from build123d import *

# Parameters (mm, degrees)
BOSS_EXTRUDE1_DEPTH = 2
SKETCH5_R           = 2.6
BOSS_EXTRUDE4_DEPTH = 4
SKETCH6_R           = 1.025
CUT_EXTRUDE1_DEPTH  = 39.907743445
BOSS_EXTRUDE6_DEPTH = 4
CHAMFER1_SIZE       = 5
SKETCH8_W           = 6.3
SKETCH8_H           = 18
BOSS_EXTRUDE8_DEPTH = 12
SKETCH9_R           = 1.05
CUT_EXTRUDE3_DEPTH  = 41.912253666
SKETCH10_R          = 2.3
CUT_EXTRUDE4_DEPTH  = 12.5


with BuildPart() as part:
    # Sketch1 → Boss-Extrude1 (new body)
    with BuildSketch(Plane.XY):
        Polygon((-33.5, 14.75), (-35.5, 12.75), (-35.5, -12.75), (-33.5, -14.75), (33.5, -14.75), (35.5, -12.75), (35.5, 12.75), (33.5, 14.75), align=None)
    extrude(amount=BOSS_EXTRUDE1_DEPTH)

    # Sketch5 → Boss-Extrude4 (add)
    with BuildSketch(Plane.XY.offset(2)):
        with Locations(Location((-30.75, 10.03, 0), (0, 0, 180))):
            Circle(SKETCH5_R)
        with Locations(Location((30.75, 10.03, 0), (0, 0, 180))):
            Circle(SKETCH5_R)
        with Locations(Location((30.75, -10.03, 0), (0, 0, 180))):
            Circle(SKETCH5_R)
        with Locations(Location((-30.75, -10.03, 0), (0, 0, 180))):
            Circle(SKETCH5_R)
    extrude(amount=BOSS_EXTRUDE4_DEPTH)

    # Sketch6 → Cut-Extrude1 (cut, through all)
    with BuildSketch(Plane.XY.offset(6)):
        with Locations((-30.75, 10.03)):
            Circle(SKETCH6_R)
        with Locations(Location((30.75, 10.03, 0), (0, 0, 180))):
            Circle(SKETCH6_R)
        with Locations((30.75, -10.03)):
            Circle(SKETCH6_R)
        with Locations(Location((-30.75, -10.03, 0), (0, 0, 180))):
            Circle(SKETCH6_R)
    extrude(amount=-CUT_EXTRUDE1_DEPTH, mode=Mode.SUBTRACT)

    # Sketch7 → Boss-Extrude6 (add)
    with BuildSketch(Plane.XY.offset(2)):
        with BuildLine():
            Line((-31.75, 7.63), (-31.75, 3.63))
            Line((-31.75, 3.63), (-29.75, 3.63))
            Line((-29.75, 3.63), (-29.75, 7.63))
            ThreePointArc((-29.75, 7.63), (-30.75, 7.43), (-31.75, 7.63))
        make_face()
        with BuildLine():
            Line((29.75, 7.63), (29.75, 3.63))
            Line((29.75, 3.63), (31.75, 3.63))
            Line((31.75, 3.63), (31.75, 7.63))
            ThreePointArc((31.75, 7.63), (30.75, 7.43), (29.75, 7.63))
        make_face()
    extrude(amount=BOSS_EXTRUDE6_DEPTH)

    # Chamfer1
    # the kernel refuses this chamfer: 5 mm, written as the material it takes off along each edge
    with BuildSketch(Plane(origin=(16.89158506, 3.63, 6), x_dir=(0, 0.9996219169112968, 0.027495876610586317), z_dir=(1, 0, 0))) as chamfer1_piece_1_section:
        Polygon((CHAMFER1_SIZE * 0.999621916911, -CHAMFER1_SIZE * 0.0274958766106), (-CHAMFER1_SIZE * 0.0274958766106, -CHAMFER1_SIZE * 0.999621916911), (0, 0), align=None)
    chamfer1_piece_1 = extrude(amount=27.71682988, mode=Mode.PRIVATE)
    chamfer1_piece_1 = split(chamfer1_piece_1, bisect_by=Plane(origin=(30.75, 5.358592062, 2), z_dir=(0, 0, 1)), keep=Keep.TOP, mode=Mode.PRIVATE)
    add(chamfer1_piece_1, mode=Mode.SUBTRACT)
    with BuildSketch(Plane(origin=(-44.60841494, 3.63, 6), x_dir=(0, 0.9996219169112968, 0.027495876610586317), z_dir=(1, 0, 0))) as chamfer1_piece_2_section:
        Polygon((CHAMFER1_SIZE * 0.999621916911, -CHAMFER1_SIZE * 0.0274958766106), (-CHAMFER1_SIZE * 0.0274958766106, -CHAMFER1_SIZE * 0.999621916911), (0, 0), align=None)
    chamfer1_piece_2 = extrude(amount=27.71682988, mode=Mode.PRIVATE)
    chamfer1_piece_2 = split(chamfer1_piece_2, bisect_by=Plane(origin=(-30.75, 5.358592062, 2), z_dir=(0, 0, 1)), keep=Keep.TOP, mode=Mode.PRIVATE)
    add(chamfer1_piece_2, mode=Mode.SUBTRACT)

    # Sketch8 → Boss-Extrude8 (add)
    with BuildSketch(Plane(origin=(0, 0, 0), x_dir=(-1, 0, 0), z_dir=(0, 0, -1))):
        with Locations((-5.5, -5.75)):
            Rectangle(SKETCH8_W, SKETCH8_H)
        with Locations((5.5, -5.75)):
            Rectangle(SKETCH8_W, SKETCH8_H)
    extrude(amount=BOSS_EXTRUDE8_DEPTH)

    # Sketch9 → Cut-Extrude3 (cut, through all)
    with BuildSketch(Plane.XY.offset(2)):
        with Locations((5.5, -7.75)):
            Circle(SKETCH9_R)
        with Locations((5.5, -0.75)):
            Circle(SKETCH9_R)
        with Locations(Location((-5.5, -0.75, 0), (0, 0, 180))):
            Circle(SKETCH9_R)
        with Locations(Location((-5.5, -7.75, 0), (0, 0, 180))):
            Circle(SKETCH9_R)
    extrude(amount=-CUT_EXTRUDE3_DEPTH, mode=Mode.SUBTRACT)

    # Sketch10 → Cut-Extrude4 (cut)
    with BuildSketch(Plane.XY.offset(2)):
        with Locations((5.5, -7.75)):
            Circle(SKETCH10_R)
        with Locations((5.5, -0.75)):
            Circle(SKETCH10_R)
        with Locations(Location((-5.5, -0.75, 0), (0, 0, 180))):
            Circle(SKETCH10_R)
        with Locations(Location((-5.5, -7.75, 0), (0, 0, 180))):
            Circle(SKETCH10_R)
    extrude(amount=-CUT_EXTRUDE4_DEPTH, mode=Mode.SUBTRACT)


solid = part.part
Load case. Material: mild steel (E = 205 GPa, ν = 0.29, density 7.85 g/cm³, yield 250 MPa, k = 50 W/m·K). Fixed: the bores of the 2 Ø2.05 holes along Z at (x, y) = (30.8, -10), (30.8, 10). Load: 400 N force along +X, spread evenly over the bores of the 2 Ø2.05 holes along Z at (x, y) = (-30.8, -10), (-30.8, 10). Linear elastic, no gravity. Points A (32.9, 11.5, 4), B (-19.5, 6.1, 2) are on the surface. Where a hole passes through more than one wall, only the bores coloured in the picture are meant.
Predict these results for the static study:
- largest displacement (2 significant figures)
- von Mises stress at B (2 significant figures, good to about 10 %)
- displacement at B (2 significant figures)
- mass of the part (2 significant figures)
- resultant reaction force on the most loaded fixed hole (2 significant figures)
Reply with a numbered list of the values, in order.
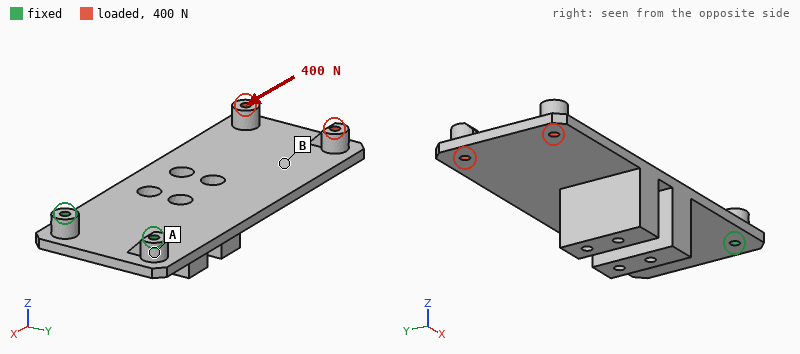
1. 0.39 mm
2. 44 MPa
3. 0.23 mm
4. 50 g
5. 200 N
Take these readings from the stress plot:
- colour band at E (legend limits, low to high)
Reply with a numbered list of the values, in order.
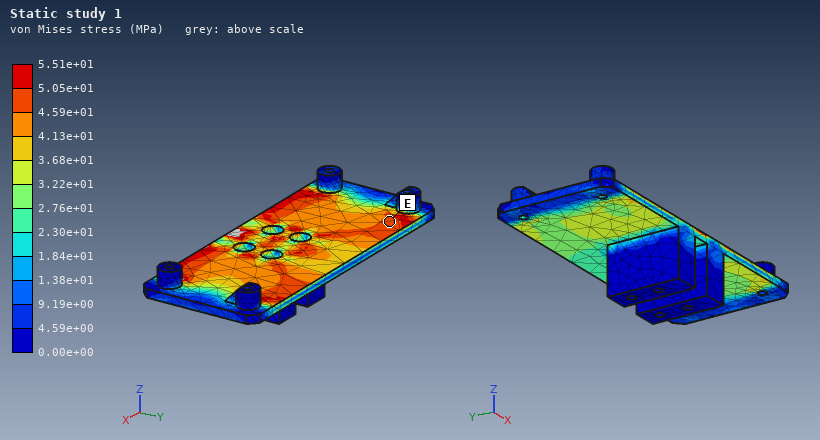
1. 4.59e+01 to 5.05e+01 MPa
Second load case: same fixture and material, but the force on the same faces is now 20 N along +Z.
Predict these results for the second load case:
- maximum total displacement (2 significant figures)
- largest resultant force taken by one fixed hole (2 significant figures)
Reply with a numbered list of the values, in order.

1. 0.39 mm
2. 10 N
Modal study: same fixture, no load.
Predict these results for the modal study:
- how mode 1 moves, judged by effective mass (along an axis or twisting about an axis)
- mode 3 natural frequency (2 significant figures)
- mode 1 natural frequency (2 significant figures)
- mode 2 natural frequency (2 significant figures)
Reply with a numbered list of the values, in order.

1. along Z
2. 2000 Hz
3. 340 Hz
4. 1600 Hz
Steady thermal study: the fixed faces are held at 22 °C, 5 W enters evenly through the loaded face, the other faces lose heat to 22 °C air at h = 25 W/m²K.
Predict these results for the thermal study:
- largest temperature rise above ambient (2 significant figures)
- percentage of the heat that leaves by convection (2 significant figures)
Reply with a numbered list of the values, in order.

1. 59 K
2. 70 %
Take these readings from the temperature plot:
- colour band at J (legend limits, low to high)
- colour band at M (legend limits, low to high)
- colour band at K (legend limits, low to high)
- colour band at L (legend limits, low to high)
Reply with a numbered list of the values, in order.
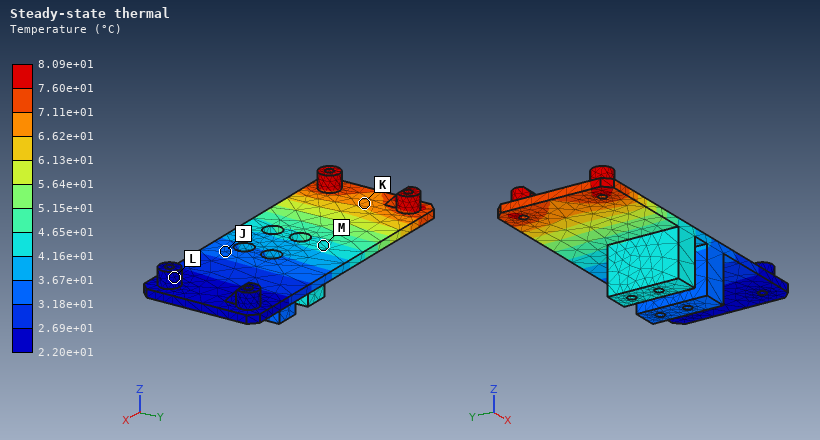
1. 3.18e+01 to 3.67e+01 °C
2. 4.16e+01 to 4.65e+01 °C
3. 6.62e+01 to 7.11e+01 °C
4. 2.20e+01 to 2.69e+01 °C
